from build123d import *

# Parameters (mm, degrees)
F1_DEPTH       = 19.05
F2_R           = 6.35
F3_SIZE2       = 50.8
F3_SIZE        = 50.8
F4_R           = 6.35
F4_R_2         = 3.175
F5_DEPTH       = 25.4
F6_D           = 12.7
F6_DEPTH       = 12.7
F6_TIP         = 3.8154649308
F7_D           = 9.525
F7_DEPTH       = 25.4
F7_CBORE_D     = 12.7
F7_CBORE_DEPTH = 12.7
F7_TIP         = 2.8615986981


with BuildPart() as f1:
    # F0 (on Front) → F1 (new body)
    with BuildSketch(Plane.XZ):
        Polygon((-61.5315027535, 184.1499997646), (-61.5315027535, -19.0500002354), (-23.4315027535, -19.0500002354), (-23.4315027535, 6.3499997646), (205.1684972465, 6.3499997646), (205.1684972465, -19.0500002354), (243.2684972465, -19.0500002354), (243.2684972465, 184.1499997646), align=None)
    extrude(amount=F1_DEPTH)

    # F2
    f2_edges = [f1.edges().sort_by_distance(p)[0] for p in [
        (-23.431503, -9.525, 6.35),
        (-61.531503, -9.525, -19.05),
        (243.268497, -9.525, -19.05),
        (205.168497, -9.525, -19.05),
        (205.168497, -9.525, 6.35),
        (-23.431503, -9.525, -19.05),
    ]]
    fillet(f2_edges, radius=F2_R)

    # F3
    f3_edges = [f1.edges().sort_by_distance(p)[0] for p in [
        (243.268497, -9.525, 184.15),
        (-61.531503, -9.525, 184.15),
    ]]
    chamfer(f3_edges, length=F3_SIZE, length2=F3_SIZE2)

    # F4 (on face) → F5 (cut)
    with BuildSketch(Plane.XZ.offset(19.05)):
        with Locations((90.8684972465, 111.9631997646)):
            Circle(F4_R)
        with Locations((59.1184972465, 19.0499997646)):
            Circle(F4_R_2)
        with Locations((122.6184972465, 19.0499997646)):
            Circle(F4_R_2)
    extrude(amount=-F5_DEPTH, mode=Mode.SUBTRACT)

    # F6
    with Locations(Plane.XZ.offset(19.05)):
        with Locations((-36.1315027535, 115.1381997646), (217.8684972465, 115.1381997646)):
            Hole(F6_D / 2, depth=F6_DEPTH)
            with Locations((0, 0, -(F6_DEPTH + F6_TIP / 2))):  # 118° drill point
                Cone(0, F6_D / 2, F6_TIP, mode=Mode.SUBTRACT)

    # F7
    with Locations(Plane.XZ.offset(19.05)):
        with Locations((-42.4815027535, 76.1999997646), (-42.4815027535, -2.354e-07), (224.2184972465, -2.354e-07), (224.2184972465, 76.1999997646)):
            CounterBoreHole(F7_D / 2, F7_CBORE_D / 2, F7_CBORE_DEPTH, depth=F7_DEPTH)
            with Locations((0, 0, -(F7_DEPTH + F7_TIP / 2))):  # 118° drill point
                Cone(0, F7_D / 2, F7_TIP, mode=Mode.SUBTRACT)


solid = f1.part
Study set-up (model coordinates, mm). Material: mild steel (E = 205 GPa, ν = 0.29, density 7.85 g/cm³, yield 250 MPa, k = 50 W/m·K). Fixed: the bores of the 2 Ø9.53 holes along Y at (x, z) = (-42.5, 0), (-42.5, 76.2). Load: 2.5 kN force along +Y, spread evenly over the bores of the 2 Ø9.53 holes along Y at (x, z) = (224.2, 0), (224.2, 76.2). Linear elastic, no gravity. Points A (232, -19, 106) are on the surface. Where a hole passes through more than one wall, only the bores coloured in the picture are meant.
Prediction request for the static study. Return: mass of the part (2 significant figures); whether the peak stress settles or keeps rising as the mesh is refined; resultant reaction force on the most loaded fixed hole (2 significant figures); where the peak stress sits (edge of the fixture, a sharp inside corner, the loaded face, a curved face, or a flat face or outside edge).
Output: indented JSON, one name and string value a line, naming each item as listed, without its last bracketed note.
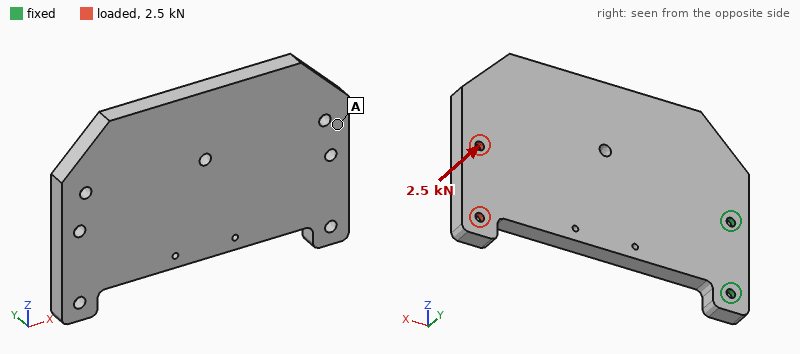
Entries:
{
  "mass of the part": "7.9 kg",
  "whether the peak stress settles or keeps rising as the mesh is refined": "keeps rising",
  "resultant reaction force on the most loaded fixed hole": "3.4 kN",
  "where the peak stress sits": "edge of the fixture"
}
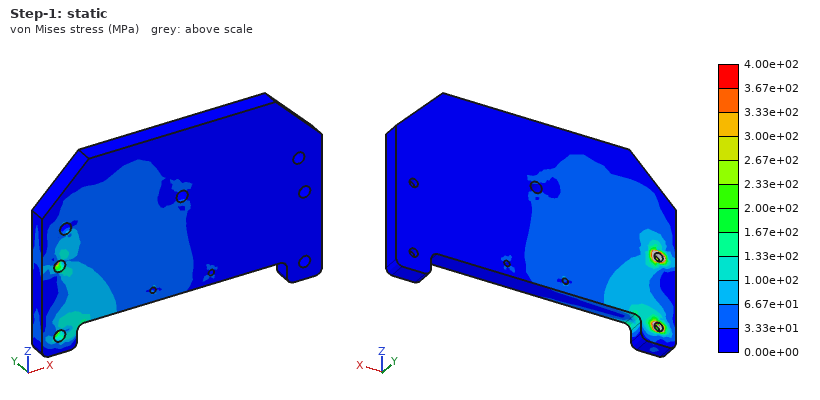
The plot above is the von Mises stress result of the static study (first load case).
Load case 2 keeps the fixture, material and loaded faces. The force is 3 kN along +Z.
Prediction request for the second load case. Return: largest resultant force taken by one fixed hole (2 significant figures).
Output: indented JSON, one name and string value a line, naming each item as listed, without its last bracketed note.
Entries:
{
  "largest resultant force taken by one fixed hole": "10 kN"
}
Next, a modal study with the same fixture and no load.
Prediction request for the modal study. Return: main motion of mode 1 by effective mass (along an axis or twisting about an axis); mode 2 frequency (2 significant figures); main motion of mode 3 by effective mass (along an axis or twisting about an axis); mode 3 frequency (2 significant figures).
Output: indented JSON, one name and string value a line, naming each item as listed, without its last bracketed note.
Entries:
{
  "main motion of mode 1 by effective mass": "along Y",
  "mode 2 frequency": "470 Hz",
  "main motion of mode 3 by effective mass": "along Z",
  "mode 3 frequency": "610 Hz"
}
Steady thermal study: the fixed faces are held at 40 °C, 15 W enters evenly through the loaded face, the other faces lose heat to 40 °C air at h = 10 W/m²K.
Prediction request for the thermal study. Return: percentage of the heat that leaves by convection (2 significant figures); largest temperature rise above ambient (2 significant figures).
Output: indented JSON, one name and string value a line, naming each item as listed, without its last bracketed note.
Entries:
{
  "percentage of the heat that leaves by convection": "67 %",
  "largest temperature rise above ambient": "25 K"
}
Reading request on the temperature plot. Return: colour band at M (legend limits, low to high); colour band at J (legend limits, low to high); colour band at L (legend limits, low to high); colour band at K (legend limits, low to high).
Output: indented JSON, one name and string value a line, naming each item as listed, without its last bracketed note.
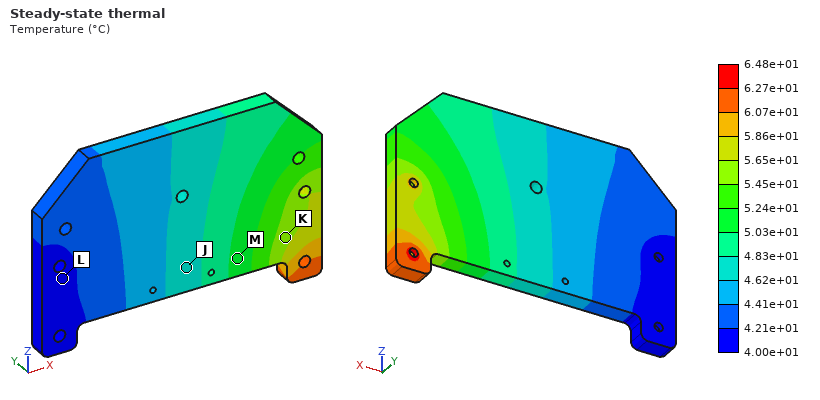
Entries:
{
  "colour band at M": "5.03e+01 to 5.24e+01 °C",
  "colour band at J": "4.62e+01 to 4.83e+01 °C",
  "colour band at L": "4.00e+01 to 4.21e+01 °C",
  "colour band at K": "5.45e+01 to 5.65e+01 °C"
}
